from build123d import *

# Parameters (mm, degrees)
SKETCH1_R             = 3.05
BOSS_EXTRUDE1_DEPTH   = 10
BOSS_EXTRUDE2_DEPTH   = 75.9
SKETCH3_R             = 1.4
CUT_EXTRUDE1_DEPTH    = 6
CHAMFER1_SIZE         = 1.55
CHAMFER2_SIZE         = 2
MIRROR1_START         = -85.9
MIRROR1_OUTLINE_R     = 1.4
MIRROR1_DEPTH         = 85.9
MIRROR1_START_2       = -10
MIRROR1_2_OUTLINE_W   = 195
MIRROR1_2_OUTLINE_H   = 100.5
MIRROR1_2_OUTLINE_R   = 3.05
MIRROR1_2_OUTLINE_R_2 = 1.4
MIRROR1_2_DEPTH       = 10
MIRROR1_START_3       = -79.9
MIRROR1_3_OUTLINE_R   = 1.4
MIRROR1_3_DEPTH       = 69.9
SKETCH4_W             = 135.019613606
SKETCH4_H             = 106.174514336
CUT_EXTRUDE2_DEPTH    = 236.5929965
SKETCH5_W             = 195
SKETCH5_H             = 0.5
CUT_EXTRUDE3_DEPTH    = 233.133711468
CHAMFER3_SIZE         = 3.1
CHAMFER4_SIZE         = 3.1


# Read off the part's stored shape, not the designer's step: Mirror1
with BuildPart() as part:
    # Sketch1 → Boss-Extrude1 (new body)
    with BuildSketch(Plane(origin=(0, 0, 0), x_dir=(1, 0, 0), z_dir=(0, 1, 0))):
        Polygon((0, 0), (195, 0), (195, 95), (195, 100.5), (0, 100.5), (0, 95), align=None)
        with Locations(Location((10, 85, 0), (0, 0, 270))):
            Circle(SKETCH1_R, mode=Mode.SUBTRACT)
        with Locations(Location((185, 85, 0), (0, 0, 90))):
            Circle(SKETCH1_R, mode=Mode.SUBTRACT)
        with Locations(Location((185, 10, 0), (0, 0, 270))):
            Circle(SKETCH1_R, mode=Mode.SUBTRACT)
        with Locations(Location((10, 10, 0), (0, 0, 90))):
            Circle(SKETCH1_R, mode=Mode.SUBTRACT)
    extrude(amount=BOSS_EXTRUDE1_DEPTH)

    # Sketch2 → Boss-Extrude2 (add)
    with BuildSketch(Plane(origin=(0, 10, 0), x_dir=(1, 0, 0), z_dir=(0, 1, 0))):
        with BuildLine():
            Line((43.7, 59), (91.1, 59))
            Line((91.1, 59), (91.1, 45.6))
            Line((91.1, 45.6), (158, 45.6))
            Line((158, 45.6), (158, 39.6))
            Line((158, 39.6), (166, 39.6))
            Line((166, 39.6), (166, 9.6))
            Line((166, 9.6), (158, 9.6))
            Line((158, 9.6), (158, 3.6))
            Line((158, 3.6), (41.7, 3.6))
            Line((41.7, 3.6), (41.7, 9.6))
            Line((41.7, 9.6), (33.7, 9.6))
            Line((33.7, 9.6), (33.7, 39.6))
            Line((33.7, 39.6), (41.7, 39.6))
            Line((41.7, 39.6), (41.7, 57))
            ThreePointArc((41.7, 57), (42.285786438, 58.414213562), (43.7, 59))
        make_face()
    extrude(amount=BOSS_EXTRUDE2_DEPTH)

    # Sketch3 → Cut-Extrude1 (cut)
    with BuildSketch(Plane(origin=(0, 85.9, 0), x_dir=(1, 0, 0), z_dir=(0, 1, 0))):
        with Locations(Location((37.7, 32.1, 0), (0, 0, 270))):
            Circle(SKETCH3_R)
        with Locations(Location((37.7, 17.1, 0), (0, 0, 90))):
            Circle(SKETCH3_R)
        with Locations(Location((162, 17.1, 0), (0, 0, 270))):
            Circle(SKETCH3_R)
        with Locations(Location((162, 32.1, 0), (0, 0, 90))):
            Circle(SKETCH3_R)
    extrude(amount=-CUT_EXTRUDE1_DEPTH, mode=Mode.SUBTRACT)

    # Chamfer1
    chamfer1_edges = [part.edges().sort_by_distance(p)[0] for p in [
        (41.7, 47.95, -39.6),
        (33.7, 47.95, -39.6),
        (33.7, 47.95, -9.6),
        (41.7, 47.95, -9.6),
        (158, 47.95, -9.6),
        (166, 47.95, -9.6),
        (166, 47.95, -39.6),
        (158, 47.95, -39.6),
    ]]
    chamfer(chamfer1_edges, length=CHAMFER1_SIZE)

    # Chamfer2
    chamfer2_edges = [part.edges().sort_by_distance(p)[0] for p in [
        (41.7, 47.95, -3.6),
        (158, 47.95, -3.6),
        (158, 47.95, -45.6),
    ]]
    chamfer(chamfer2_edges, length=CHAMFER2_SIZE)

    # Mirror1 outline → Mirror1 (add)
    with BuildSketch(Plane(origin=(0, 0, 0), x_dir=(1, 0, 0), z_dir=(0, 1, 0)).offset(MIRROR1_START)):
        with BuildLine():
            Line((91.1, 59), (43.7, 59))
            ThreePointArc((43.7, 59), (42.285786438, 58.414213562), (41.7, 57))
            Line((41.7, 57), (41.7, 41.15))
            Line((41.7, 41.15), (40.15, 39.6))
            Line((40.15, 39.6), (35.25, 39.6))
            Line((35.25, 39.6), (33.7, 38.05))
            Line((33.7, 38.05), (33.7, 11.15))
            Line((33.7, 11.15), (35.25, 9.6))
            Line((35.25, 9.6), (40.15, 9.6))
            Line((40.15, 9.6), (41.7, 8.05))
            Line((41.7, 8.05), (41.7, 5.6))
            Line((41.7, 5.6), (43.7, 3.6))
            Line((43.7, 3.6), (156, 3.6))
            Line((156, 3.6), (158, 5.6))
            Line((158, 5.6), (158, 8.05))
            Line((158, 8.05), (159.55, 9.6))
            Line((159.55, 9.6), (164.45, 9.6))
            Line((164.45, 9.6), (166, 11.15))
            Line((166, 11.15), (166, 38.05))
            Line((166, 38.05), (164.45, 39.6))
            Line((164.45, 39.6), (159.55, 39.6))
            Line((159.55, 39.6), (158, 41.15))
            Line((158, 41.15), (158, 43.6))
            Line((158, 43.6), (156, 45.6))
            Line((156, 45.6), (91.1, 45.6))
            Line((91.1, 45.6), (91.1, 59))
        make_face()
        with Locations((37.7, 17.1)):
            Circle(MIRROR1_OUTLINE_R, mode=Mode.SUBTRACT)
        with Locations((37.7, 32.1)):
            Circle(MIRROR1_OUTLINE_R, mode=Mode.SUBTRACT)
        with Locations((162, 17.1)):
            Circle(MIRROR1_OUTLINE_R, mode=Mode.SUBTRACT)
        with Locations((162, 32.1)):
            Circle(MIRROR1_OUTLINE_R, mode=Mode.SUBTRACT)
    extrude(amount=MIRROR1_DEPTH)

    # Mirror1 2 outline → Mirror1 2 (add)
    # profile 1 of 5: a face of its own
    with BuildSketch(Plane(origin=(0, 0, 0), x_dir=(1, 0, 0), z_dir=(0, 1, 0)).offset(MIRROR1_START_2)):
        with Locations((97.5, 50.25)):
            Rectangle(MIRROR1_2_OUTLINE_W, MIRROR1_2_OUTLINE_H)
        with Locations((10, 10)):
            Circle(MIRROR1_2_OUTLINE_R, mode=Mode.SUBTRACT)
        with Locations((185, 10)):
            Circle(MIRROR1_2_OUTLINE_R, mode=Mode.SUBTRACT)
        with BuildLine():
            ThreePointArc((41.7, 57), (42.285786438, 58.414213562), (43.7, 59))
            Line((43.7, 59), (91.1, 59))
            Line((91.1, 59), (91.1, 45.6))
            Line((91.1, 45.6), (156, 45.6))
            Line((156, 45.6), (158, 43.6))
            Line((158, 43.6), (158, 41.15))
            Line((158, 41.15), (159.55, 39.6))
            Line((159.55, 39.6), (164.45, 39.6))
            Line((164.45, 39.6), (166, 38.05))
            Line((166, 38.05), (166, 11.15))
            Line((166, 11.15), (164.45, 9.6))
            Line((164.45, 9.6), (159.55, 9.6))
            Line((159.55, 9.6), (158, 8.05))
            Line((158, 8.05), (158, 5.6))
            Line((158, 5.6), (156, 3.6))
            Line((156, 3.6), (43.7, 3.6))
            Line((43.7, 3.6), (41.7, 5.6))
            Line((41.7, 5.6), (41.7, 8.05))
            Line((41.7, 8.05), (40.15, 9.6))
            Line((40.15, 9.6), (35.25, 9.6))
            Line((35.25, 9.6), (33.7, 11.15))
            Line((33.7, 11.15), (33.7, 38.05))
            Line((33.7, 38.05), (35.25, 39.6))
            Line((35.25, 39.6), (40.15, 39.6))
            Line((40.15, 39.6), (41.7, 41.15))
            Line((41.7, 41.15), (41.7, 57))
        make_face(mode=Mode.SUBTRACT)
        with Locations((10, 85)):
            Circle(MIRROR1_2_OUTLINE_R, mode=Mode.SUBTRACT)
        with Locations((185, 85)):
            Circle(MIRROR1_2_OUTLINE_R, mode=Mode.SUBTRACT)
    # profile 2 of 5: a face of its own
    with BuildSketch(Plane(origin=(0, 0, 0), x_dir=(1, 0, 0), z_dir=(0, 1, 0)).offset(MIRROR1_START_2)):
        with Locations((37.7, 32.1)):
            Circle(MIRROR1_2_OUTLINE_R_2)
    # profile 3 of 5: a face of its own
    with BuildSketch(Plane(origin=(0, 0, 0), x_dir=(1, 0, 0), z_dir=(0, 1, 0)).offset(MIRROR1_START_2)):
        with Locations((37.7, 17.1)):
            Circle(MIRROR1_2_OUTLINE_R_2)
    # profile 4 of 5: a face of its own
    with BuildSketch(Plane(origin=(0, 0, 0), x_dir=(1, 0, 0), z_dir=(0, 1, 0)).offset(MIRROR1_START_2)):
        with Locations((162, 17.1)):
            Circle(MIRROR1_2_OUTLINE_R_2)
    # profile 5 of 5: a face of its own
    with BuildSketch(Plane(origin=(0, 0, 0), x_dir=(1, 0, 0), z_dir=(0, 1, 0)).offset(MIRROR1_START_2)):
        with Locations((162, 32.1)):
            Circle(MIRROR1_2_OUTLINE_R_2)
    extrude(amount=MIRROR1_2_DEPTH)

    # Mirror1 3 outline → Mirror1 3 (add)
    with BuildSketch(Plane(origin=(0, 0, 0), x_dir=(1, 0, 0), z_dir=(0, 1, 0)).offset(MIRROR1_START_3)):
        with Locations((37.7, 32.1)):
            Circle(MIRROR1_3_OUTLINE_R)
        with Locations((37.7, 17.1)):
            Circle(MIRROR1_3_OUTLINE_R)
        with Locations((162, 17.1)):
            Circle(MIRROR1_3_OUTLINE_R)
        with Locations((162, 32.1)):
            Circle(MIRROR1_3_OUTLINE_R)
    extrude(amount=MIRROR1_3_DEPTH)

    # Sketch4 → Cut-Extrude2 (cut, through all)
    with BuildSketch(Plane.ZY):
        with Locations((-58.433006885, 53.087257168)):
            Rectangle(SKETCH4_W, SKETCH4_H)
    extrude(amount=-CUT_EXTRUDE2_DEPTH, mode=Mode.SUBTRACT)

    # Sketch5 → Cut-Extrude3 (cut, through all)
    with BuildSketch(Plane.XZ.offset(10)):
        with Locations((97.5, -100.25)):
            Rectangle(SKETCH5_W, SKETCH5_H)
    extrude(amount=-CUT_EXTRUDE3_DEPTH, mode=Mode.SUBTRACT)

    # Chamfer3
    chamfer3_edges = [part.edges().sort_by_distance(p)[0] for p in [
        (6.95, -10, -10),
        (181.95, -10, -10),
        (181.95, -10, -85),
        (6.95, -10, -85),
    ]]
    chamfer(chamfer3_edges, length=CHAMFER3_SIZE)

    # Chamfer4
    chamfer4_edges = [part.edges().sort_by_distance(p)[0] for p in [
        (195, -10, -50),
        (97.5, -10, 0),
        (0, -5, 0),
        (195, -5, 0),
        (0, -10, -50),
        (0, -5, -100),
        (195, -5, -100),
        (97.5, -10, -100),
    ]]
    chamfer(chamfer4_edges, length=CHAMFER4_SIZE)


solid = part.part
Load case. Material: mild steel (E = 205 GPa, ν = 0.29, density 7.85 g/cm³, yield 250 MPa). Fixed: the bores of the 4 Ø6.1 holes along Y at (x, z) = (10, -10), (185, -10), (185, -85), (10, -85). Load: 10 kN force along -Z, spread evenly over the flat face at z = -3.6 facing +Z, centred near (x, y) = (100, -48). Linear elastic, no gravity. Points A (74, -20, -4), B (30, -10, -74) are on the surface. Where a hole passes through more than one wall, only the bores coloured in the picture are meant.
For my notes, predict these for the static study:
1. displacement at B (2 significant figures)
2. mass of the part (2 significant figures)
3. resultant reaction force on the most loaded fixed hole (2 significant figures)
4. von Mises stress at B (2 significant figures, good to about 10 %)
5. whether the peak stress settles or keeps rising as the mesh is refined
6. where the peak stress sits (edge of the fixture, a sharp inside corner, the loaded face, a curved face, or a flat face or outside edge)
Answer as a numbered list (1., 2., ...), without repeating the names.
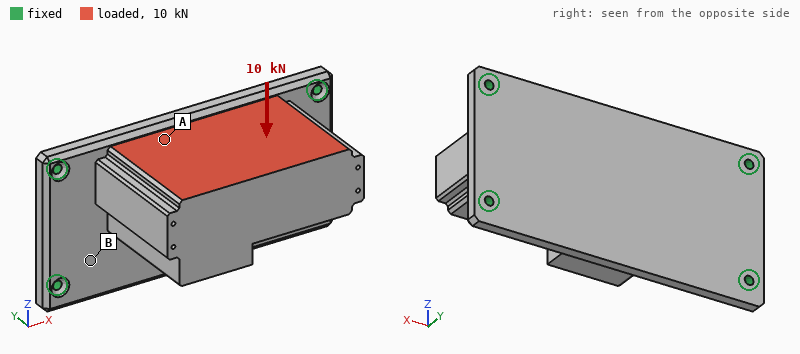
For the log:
1. 0.025 mm
2. 5.1 kg
3. 5.2 kN
4. 38 MPa
5. keeps rising
6. edge of the fixture
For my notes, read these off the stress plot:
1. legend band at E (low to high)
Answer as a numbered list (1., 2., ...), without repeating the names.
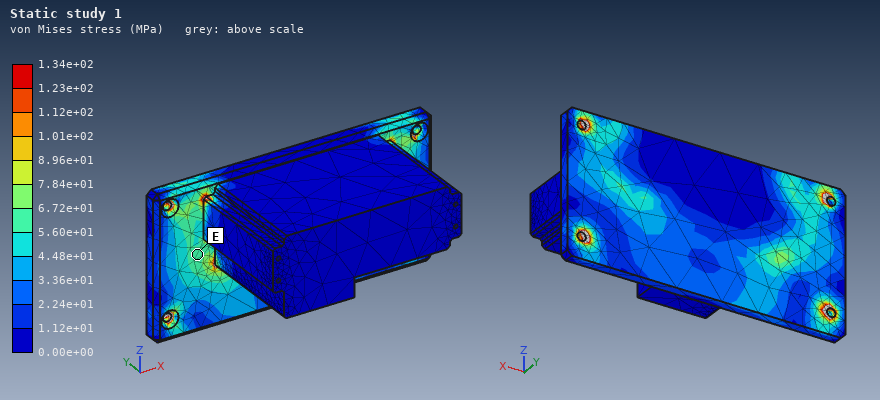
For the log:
1. 5.60e+01 to 6.72e+01 MPa
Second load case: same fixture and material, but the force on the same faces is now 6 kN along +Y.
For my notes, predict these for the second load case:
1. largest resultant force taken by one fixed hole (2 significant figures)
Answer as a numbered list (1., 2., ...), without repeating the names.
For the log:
1. 4.0 kN
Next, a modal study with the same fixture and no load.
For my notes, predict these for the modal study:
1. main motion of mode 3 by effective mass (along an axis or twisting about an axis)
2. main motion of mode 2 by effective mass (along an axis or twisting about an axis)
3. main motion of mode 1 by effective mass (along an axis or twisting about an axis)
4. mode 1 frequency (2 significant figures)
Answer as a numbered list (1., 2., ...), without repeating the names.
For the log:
1. along X
2. along Y
3. along Z
4. 870 Hz
